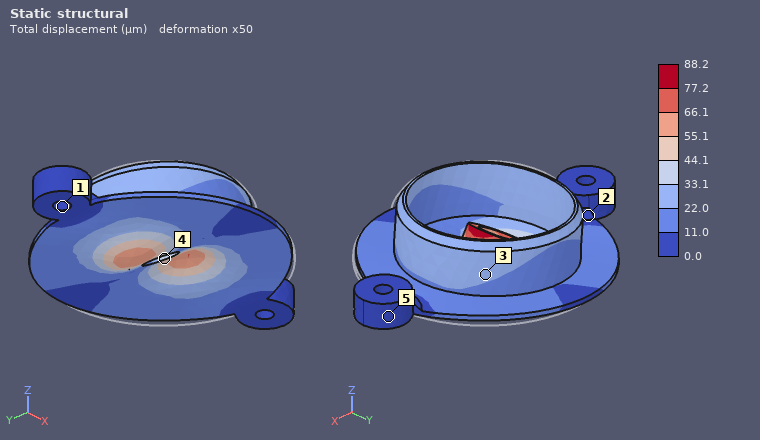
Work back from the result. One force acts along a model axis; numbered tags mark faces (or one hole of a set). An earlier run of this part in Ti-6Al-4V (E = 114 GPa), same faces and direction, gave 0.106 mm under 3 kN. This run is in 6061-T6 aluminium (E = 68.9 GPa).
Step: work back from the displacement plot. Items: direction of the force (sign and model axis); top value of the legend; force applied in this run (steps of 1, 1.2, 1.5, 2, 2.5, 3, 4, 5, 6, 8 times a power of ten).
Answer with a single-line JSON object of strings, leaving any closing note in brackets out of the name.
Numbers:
{"direction of the force": "-X", "top value of the legend": "88.2 µm", "force applied in this run": "1.5 kN"}
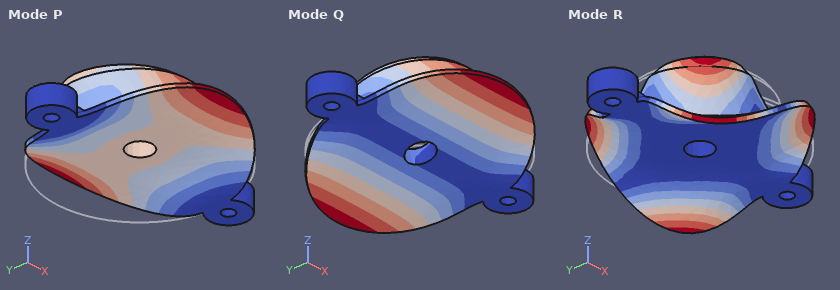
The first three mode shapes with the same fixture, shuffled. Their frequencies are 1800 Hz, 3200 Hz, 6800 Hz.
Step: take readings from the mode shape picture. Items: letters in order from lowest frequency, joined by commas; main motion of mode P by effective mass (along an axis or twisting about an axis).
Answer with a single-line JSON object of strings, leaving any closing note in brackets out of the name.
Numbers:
{"letters in order from lowest frequency, joined by commas": "Q, P, R", "main motion of mode P by effective mass": "along Z"}
